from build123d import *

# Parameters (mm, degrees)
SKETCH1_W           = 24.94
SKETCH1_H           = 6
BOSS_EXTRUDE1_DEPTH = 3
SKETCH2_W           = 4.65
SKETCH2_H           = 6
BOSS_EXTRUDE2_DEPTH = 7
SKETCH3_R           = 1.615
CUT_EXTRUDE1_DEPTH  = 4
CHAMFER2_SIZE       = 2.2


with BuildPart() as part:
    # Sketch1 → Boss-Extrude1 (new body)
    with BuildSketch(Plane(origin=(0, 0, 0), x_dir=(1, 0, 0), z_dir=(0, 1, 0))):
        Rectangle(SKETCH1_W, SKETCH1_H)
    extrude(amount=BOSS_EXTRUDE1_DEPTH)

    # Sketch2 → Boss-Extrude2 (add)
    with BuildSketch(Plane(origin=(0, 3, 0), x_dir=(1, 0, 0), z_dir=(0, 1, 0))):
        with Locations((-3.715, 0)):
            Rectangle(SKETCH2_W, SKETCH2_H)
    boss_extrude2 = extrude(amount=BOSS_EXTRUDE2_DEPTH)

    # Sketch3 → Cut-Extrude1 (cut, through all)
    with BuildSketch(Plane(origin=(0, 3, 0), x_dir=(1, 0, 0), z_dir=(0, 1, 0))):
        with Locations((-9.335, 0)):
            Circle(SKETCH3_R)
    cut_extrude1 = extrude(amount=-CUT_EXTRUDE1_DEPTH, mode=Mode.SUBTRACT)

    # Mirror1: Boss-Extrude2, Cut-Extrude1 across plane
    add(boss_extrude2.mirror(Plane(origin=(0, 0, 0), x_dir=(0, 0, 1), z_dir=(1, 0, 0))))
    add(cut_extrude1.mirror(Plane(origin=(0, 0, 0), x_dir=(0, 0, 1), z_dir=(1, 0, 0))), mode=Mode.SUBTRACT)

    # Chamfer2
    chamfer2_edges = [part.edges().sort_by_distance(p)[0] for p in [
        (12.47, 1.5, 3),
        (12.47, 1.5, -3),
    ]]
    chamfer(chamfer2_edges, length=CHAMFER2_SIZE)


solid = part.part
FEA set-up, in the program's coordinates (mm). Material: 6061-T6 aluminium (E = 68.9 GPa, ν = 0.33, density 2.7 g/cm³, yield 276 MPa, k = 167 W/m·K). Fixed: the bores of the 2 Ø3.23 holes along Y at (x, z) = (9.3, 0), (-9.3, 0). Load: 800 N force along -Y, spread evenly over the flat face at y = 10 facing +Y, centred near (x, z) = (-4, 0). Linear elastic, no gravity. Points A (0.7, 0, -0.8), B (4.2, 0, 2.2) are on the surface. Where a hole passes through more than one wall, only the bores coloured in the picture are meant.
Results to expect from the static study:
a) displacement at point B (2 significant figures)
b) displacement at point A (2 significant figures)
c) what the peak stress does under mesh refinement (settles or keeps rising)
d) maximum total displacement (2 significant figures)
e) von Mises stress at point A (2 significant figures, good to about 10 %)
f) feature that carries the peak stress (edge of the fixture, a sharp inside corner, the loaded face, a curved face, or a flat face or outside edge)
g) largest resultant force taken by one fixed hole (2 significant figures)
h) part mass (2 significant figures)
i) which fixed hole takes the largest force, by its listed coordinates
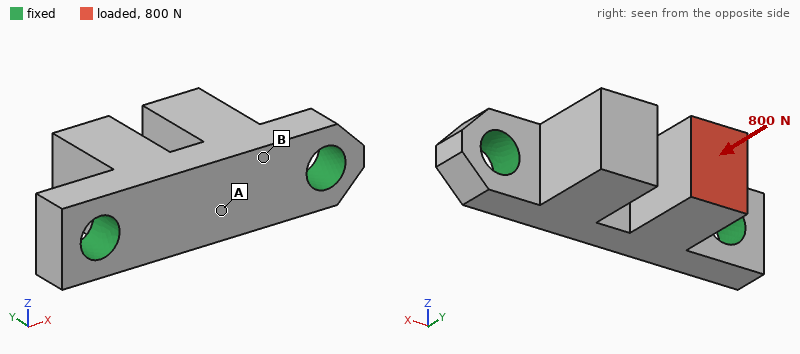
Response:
7.4 µm
14 µm
keeps rising
26 µm
55 MPa
edge of the fixture
630 N
2.1 g
(-9.3, 0)
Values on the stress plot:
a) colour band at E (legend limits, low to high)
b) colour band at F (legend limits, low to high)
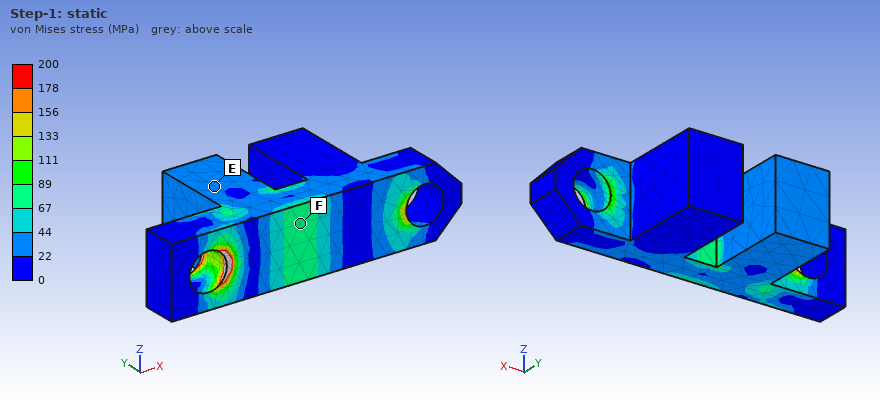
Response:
22 to 44 MPa
67 to 89 MPa
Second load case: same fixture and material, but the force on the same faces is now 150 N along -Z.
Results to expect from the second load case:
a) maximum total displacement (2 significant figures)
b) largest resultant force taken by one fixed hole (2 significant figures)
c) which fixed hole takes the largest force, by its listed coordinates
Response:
28 µm
120 N
(-9.3, 0)
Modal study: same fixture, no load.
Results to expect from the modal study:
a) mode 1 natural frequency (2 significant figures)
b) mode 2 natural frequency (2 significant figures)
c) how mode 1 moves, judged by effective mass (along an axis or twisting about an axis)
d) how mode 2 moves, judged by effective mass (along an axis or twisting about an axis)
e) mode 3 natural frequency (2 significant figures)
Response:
21 kHz
23 kHz
along Z
along Y
31 kHz
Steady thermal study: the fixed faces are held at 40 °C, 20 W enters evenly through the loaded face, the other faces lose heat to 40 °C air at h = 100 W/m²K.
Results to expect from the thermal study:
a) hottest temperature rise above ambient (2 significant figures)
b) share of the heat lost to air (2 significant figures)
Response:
48 K
4.2 %
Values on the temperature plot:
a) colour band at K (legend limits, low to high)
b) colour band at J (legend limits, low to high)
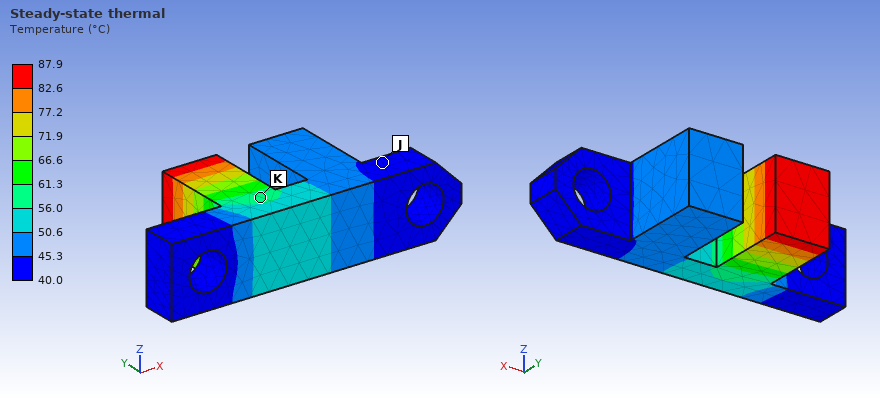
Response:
56.0 to 61.3 °C
40.0 to 45.3 °C
